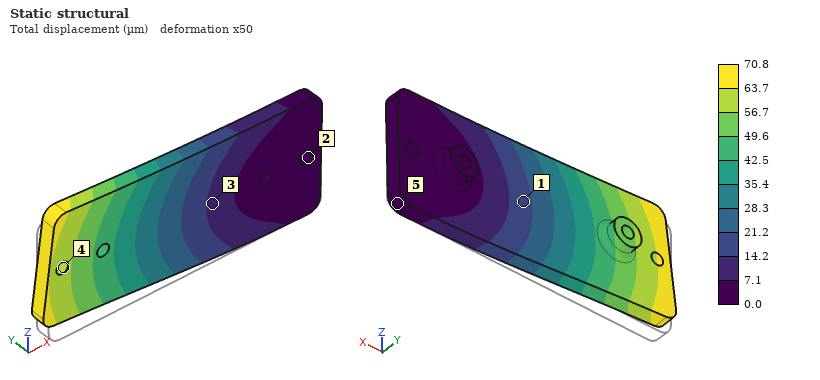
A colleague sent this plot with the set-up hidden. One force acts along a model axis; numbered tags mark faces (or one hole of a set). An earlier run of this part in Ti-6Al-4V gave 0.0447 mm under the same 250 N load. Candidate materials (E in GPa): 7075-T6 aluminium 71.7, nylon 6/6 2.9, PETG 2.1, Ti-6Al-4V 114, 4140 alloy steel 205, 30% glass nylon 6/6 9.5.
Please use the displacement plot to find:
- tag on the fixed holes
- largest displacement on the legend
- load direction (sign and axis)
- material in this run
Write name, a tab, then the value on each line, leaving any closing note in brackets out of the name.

tag on the fixed holes	2
largest displacement on the legend	70.8 µm
load direction	+Z
material in this run	7075-T6 aluminium
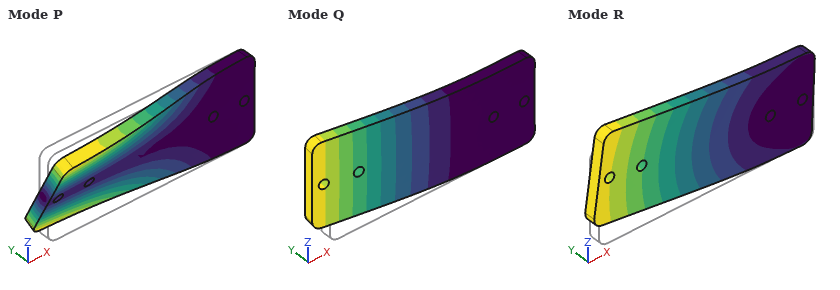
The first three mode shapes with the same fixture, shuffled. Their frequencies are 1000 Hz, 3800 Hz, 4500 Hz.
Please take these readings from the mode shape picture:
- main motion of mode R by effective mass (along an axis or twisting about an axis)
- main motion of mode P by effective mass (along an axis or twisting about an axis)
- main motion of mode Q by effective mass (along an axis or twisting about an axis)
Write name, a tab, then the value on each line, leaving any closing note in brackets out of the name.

main motion of mode R by effective mass	along Z
main motion of mode P by effective mass	twisting about X
main motion of mode Q by effective mass	along Y
